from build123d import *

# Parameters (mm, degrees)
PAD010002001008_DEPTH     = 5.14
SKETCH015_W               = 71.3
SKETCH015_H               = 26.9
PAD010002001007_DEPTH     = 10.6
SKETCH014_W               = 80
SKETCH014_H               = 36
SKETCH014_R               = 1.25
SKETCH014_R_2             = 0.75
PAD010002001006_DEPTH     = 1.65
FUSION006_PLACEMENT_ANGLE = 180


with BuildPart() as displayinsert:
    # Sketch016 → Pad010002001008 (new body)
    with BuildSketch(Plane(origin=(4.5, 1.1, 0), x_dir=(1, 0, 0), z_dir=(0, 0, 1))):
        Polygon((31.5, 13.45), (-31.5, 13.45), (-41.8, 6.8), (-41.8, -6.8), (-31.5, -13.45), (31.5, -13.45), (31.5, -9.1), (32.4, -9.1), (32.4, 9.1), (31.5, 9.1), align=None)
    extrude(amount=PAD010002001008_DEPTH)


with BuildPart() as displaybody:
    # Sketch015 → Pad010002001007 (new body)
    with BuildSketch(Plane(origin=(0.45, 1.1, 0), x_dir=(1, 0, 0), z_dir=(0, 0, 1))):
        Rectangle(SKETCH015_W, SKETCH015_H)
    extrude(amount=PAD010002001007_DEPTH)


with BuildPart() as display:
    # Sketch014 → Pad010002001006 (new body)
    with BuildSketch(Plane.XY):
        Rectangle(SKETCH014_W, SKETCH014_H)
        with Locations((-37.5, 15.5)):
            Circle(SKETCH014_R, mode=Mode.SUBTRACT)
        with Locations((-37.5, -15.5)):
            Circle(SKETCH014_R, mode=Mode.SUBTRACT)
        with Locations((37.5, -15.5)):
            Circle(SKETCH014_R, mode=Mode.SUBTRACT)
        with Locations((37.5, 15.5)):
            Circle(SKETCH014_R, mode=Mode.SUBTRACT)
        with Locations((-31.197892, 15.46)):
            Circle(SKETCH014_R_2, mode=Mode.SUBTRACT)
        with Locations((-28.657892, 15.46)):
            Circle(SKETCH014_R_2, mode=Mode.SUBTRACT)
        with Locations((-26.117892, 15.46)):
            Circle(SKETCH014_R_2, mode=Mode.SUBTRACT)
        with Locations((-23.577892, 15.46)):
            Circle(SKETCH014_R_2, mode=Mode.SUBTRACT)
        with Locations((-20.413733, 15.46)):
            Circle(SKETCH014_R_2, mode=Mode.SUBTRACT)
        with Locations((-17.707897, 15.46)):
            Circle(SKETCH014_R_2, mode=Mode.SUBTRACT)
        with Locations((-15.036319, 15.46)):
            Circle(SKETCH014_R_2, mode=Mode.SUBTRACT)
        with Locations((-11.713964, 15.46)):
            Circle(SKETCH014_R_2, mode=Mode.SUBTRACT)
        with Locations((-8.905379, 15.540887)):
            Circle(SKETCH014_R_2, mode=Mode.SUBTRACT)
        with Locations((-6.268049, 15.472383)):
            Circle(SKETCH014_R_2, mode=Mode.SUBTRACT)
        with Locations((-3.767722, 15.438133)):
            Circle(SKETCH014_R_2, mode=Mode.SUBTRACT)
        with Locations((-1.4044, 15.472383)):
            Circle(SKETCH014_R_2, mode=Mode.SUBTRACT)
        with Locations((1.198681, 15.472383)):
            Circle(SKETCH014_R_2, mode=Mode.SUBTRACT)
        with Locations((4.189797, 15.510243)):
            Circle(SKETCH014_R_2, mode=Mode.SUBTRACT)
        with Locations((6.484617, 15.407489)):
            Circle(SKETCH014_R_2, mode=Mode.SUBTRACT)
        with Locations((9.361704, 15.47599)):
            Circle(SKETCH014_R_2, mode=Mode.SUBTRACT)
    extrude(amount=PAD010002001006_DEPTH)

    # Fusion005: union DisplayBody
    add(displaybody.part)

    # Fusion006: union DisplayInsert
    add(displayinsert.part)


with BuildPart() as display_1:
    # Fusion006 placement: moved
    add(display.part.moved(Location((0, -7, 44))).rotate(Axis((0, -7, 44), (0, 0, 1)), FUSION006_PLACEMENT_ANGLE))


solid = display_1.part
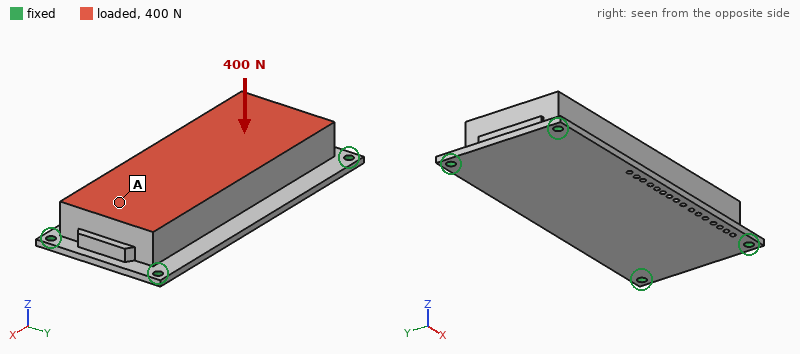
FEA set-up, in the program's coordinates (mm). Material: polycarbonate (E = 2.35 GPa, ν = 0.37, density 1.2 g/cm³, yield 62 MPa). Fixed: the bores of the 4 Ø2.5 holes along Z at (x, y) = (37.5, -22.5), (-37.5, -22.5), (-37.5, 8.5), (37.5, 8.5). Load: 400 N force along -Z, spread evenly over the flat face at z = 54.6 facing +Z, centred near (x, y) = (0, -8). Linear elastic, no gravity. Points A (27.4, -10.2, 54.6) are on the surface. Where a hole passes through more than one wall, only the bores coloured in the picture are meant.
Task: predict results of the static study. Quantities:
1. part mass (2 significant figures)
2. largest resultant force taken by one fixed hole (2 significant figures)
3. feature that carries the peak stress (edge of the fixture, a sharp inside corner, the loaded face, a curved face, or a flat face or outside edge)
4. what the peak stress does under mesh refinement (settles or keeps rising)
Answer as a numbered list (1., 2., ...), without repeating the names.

1. 26 g
2. 170 N
3. edge of the fixture
4. keeps rising
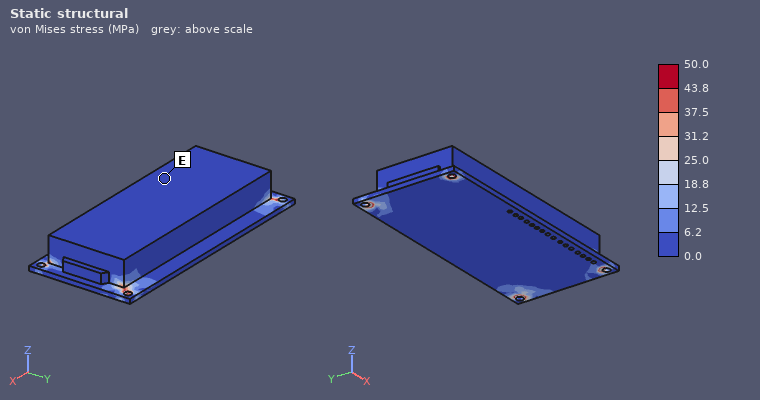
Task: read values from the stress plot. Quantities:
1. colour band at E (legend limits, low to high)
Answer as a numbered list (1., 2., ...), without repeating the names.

1. 0.0 to 6.2 MPa
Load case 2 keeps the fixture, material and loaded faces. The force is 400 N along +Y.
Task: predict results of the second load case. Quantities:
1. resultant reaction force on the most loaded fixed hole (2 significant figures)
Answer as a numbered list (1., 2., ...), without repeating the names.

1. 150 N
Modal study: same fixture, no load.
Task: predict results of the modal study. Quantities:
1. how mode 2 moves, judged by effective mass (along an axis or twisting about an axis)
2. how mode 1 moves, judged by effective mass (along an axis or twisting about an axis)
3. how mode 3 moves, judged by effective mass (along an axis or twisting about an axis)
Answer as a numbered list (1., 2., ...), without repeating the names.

1. along Y
2. along Z
3. twisting about Y
